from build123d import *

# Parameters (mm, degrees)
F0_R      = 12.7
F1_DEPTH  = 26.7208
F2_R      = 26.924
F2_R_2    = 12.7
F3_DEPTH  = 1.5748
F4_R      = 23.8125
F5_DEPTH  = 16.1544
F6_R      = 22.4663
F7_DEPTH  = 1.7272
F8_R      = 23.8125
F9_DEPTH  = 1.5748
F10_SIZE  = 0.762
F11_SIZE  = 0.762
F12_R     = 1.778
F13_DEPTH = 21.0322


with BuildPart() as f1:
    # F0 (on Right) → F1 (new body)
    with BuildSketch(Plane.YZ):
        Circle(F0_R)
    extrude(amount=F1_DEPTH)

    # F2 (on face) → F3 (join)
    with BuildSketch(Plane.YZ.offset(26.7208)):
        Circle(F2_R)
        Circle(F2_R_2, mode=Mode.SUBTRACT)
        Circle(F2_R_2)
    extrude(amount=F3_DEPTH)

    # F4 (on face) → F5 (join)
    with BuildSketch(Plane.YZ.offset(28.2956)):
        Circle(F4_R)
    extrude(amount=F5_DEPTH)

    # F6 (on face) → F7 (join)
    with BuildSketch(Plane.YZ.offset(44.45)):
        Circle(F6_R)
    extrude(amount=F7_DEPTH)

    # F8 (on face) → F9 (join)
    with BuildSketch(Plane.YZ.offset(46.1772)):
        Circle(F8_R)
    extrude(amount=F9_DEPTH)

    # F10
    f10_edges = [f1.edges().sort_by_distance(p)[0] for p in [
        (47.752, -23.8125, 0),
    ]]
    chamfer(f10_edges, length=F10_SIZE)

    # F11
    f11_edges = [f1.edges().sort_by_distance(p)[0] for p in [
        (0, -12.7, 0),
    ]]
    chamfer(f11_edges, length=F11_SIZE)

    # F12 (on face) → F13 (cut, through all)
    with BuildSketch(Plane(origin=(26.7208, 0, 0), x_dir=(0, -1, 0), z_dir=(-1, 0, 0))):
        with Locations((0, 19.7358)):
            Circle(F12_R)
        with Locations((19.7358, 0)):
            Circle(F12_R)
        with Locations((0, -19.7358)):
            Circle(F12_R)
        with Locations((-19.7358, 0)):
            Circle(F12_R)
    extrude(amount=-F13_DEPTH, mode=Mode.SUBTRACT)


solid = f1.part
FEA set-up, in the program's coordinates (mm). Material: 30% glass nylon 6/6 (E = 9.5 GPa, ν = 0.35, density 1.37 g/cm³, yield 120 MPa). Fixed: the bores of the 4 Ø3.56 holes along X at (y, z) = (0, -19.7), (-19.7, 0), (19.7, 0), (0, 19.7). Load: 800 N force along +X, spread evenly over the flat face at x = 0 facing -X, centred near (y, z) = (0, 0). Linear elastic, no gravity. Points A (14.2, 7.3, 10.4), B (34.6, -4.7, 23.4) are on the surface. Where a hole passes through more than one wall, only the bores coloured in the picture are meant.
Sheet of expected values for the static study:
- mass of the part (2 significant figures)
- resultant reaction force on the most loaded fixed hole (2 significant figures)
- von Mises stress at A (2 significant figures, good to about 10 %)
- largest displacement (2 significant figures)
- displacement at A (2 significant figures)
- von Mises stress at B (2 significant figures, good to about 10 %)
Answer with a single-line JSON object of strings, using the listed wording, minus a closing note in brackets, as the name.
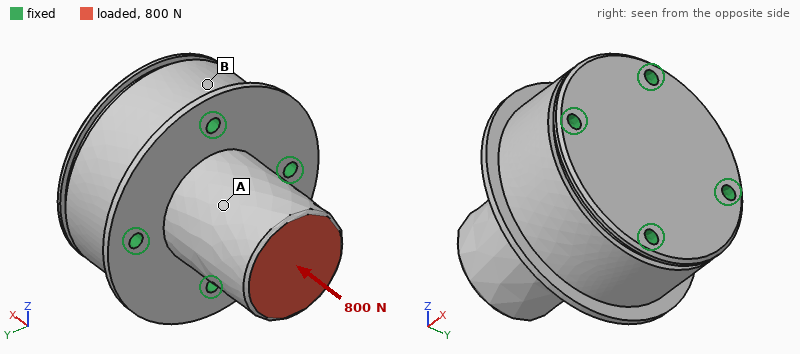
{"mass of the part": "69 g", "resultant reaction force on the most loaded fixed hole": "210 N", "von Mises stress at A": "1.5 MPa", "largest displacement": "7.1 µm", "displacement at A": "4.6 µm", "von Mises stress at B": "0.45 MPa"}
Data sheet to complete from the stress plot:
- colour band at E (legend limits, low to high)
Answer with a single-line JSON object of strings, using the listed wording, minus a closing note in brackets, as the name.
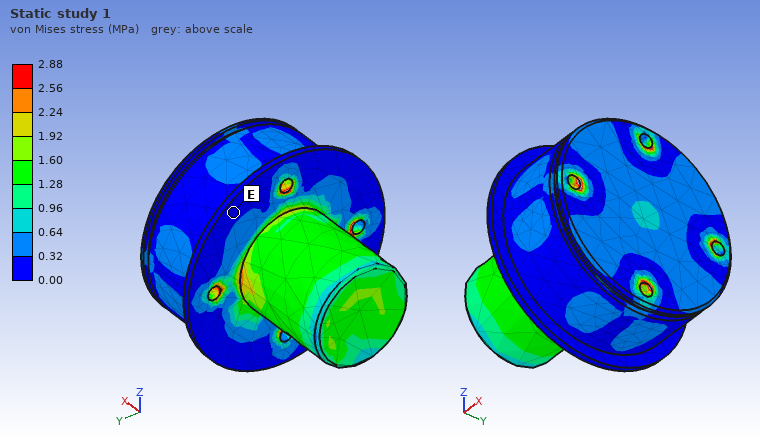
{"colour band at E": "0.00 to 0.32 MPa"}
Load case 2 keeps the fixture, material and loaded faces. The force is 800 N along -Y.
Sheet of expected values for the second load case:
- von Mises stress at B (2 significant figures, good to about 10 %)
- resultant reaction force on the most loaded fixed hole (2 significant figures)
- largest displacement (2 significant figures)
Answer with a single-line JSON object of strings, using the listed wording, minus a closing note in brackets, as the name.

{"von Mises stress at B": "1.1 MPa", "resultant reaction force on the most loaded fixed hole": "700 N", "largest displacement": "68 µm"}
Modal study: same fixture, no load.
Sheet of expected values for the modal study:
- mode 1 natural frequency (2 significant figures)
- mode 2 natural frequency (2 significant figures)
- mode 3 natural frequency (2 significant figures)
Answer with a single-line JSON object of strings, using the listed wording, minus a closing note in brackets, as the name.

{"mode 1 natural frequency": "7000 Hz", "mode 2 natural frequency": "7000 Hz", "mode 3 natural frequency": "13 kHz"}
